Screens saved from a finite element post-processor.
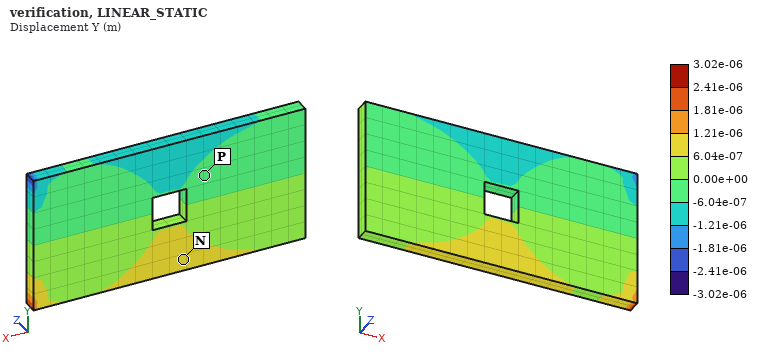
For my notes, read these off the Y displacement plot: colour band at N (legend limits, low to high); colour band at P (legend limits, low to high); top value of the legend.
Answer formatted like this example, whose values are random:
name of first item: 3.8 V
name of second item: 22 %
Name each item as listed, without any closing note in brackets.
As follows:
colour band at N: 6.04e-07 to 1.21e-06 m
colour band at P: -6.04e-07 to 0.00e+00 m
top value of the legend: 3.02e-06 m
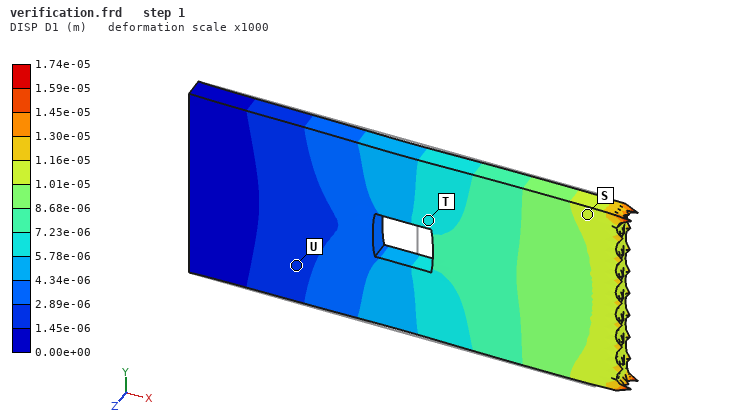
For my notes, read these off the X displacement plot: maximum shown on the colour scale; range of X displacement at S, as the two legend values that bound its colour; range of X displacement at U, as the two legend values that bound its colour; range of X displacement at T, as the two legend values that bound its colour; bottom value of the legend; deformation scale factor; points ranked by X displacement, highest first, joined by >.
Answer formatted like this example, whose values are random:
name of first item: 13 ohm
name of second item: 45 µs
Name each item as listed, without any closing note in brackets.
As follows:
maximum shown on the colour scale: 1.74e-05 m
range of X displacement at S, as the two legend values that bound its colour: 1.01e-05 to 1.16e-05 m
range of X displacement at U, as the two legend values that bound its colour: 1.45e-06 to 2.89e-06 m
range of X displacement at T, as the two legend values that bound its colour: 5.78e-06 to 7.23e-06 m
bottom value of the legend: 0.00e+00 m
deformation scale factor: 1000
points ranked by X displacement, highest first, joined by >: S > T > U
